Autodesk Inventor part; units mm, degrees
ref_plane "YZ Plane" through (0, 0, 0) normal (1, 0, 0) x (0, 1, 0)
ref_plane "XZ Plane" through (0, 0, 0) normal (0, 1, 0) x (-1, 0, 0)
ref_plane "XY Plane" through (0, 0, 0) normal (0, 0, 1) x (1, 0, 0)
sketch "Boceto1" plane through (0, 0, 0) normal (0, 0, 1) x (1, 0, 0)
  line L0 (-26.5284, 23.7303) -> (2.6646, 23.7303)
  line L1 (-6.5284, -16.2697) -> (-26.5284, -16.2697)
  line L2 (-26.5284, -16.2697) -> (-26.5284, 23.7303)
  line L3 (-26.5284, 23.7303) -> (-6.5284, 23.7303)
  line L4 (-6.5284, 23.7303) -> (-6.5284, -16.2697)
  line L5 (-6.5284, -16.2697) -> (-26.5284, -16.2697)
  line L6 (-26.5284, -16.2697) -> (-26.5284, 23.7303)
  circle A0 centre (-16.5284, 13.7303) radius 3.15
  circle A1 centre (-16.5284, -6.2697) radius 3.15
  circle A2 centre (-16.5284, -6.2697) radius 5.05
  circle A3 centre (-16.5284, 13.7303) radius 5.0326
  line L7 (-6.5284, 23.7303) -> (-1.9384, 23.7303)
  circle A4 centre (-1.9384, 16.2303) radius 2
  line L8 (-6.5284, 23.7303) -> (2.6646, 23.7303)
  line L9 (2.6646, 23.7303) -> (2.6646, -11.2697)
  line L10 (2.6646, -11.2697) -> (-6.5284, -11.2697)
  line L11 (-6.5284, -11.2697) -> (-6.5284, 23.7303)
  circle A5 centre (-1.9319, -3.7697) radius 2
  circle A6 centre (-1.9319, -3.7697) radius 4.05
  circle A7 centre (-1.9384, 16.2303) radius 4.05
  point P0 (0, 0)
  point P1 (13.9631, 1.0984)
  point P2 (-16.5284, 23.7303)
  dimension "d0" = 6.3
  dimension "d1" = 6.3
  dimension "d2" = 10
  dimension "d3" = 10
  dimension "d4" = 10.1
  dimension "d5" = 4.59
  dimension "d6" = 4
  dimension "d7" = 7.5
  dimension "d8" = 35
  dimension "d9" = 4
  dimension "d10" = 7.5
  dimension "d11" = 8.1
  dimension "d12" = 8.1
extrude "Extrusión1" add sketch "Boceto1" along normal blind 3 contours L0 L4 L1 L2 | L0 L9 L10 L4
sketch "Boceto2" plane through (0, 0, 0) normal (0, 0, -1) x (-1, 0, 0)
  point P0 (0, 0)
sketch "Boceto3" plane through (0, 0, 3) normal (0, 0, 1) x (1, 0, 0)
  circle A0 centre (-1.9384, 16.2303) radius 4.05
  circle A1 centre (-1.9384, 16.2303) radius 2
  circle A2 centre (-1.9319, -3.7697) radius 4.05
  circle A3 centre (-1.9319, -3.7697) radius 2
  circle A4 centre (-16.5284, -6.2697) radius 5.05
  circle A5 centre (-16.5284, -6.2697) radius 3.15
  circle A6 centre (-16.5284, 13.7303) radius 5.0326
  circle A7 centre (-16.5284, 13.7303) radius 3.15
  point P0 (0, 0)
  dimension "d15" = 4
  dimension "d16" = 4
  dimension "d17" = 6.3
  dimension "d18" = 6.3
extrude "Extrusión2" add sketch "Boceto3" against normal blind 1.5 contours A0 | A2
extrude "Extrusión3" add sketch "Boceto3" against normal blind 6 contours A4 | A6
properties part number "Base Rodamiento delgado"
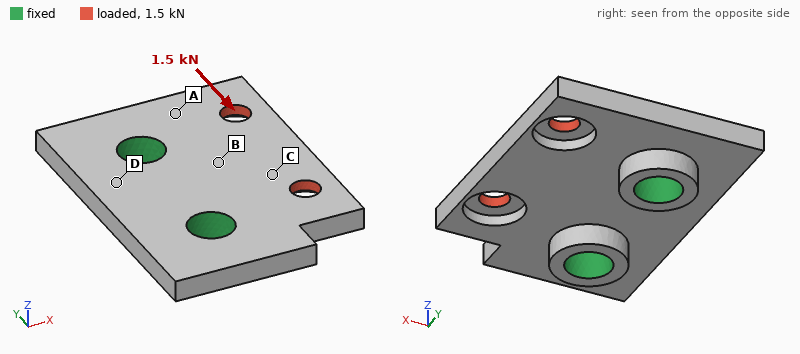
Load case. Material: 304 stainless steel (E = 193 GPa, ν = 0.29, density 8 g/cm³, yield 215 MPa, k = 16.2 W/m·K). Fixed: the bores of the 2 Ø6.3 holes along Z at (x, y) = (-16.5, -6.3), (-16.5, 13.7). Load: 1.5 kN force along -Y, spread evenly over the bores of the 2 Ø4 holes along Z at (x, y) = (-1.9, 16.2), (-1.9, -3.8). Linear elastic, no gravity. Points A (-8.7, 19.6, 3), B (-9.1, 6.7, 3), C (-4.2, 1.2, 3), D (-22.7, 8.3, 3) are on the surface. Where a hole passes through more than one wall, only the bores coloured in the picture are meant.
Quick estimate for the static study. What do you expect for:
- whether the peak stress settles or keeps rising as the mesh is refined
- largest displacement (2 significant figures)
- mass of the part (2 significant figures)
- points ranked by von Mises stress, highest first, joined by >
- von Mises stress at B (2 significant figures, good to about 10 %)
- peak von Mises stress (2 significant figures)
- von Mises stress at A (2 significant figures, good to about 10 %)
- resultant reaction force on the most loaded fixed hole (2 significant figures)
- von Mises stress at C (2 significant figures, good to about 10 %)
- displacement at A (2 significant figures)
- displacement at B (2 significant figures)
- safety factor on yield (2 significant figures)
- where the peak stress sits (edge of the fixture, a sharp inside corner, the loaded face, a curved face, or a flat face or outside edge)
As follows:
settles
8.2 µm
26 g
C > B > A > D
32 MPa
100 MPa
21 MPa
1.1 kN
45 MPa
2.5 µm
1.4 µm
2.1
the loaded face
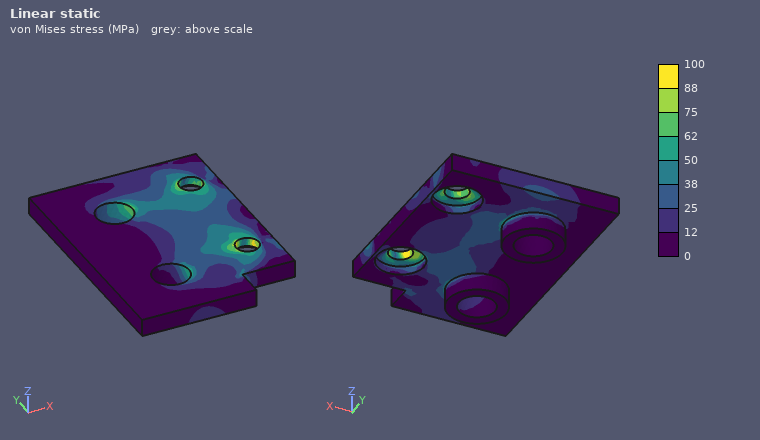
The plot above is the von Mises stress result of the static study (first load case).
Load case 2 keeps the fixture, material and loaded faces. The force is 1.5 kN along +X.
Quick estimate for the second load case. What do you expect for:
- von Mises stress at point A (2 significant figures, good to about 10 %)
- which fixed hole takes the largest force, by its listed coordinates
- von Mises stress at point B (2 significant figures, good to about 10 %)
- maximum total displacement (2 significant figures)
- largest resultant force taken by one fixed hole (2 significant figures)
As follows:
37 MPa
(-16.5, 13.7)
24 MPa
9.6 µm
900 N
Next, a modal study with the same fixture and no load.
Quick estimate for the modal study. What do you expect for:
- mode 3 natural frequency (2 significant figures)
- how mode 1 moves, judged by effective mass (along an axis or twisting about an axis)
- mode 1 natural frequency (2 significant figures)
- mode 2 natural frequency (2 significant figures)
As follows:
19 kHz
along Z
9300 Hz
13 kHz
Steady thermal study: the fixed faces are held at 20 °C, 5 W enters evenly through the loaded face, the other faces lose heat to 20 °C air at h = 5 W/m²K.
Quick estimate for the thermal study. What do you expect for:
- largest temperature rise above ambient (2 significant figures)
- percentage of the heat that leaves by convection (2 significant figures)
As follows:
60 K
4.1 %
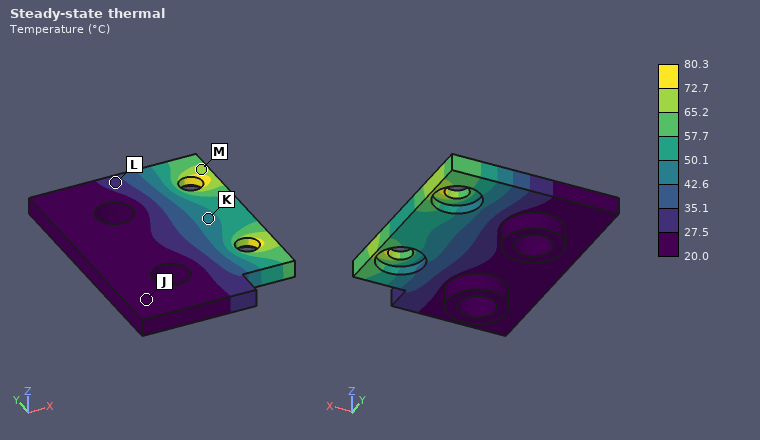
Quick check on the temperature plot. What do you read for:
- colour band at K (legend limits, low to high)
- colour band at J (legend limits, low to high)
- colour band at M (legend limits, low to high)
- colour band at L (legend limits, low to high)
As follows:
42.6 to 50.1 °C
20.0 to 27.5 °C
65.2 to 72.7 °C
27.5 to 35.1 °C
